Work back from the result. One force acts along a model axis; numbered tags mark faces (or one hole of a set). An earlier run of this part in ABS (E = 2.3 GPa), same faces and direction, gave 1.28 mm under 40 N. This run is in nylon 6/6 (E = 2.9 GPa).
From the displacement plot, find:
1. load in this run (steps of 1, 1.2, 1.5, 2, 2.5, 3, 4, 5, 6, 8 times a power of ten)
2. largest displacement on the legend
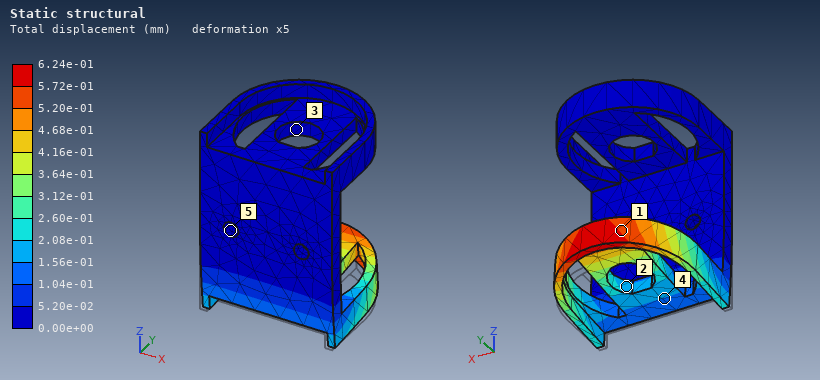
25 N
6.24e-01 mm
